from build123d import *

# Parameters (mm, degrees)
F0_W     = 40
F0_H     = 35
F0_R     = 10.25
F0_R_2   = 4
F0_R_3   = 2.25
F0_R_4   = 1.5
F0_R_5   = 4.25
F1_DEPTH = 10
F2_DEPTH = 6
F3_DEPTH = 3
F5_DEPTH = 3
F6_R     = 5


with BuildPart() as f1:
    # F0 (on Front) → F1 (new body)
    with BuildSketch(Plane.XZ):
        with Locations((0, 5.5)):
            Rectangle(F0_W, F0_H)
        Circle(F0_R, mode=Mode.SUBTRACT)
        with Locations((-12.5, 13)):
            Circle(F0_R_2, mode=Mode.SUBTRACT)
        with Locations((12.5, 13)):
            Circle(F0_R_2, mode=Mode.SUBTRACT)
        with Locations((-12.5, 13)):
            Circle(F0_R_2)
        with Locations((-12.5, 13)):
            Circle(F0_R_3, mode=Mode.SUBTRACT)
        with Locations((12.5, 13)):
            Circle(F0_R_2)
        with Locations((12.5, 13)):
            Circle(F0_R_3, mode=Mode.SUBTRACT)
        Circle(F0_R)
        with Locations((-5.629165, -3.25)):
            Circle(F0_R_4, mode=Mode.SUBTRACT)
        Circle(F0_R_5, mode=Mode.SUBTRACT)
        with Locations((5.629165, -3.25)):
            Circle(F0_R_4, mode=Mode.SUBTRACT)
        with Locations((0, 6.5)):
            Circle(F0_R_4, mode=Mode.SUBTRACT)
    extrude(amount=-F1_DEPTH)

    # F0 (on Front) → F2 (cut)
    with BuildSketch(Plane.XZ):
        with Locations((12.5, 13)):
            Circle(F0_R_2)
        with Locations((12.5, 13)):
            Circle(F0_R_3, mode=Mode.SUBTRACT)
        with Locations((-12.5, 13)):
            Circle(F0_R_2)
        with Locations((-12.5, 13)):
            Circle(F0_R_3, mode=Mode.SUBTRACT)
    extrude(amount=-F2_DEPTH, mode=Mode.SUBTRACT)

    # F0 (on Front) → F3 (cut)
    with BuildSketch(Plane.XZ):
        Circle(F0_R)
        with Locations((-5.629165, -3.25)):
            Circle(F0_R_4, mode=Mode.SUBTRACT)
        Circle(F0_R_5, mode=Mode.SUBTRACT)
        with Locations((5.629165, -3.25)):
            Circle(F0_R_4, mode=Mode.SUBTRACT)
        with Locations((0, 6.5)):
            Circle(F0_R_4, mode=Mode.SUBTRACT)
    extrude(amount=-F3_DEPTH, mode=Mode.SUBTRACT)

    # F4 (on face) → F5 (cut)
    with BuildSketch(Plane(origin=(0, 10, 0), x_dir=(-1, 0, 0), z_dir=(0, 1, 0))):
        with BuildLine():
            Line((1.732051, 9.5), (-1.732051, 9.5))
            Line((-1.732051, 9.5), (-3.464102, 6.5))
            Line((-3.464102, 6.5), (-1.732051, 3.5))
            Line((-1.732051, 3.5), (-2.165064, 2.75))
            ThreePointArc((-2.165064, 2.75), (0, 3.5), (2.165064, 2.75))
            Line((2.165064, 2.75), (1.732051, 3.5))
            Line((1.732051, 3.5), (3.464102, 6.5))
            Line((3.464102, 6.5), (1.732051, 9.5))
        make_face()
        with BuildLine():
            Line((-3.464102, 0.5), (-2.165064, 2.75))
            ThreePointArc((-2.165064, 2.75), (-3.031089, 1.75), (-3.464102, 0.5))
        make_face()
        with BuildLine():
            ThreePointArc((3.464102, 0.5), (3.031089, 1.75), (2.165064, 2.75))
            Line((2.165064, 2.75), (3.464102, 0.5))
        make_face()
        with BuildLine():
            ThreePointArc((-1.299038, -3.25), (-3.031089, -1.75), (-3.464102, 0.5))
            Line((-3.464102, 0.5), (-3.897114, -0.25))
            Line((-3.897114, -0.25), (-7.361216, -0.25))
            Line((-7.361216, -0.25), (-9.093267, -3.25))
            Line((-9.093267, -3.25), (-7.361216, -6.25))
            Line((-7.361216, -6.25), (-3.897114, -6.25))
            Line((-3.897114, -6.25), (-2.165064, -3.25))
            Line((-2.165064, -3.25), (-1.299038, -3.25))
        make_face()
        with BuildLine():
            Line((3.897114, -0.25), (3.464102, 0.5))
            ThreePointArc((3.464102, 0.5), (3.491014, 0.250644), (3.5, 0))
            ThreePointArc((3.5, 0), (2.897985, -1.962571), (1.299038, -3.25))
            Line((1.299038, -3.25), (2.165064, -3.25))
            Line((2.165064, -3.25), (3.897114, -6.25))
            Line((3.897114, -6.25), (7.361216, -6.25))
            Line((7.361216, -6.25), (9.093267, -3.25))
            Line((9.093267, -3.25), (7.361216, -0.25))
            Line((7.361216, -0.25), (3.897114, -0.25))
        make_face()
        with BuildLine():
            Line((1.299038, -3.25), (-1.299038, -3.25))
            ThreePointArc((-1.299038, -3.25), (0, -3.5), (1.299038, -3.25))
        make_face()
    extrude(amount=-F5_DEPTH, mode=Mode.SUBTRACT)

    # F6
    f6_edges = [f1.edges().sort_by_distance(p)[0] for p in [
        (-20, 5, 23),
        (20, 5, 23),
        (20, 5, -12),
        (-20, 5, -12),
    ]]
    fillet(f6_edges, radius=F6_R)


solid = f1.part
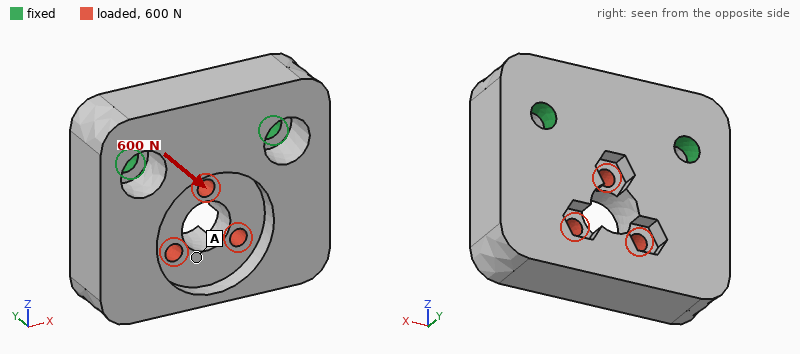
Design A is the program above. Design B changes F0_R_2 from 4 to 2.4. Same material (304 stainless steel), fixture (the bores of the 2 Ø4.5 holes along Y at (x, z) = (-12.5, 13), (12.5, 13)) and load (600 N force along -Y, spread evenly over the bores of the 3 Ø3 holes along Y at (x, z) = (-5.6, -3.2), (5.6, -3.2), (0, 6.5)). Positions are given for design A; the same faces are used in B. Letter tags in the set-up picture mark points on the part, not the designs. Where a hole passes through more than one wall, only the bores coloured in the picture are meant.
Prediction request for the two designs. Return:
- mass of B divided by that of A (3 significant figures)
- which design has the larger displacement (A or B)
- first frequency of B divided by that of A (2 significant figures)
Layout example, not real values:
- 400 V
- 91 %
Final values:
- 1.03
- A
- 1.1
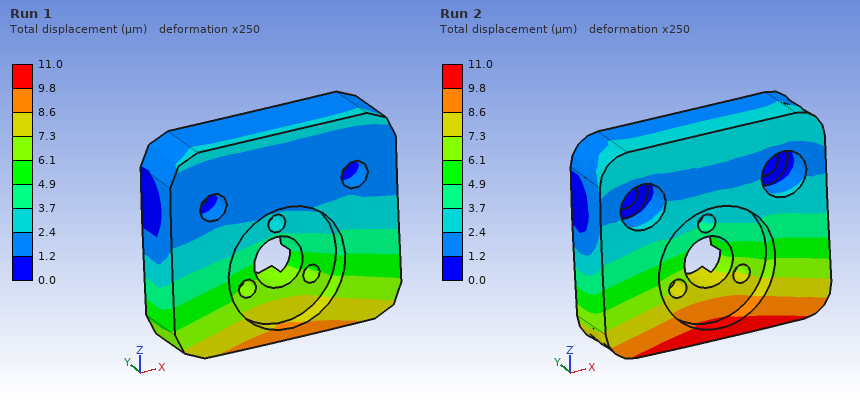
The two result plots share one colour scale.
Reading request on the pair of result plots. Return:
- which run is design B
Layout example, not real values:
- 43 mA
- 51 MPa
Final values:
- Run 1
